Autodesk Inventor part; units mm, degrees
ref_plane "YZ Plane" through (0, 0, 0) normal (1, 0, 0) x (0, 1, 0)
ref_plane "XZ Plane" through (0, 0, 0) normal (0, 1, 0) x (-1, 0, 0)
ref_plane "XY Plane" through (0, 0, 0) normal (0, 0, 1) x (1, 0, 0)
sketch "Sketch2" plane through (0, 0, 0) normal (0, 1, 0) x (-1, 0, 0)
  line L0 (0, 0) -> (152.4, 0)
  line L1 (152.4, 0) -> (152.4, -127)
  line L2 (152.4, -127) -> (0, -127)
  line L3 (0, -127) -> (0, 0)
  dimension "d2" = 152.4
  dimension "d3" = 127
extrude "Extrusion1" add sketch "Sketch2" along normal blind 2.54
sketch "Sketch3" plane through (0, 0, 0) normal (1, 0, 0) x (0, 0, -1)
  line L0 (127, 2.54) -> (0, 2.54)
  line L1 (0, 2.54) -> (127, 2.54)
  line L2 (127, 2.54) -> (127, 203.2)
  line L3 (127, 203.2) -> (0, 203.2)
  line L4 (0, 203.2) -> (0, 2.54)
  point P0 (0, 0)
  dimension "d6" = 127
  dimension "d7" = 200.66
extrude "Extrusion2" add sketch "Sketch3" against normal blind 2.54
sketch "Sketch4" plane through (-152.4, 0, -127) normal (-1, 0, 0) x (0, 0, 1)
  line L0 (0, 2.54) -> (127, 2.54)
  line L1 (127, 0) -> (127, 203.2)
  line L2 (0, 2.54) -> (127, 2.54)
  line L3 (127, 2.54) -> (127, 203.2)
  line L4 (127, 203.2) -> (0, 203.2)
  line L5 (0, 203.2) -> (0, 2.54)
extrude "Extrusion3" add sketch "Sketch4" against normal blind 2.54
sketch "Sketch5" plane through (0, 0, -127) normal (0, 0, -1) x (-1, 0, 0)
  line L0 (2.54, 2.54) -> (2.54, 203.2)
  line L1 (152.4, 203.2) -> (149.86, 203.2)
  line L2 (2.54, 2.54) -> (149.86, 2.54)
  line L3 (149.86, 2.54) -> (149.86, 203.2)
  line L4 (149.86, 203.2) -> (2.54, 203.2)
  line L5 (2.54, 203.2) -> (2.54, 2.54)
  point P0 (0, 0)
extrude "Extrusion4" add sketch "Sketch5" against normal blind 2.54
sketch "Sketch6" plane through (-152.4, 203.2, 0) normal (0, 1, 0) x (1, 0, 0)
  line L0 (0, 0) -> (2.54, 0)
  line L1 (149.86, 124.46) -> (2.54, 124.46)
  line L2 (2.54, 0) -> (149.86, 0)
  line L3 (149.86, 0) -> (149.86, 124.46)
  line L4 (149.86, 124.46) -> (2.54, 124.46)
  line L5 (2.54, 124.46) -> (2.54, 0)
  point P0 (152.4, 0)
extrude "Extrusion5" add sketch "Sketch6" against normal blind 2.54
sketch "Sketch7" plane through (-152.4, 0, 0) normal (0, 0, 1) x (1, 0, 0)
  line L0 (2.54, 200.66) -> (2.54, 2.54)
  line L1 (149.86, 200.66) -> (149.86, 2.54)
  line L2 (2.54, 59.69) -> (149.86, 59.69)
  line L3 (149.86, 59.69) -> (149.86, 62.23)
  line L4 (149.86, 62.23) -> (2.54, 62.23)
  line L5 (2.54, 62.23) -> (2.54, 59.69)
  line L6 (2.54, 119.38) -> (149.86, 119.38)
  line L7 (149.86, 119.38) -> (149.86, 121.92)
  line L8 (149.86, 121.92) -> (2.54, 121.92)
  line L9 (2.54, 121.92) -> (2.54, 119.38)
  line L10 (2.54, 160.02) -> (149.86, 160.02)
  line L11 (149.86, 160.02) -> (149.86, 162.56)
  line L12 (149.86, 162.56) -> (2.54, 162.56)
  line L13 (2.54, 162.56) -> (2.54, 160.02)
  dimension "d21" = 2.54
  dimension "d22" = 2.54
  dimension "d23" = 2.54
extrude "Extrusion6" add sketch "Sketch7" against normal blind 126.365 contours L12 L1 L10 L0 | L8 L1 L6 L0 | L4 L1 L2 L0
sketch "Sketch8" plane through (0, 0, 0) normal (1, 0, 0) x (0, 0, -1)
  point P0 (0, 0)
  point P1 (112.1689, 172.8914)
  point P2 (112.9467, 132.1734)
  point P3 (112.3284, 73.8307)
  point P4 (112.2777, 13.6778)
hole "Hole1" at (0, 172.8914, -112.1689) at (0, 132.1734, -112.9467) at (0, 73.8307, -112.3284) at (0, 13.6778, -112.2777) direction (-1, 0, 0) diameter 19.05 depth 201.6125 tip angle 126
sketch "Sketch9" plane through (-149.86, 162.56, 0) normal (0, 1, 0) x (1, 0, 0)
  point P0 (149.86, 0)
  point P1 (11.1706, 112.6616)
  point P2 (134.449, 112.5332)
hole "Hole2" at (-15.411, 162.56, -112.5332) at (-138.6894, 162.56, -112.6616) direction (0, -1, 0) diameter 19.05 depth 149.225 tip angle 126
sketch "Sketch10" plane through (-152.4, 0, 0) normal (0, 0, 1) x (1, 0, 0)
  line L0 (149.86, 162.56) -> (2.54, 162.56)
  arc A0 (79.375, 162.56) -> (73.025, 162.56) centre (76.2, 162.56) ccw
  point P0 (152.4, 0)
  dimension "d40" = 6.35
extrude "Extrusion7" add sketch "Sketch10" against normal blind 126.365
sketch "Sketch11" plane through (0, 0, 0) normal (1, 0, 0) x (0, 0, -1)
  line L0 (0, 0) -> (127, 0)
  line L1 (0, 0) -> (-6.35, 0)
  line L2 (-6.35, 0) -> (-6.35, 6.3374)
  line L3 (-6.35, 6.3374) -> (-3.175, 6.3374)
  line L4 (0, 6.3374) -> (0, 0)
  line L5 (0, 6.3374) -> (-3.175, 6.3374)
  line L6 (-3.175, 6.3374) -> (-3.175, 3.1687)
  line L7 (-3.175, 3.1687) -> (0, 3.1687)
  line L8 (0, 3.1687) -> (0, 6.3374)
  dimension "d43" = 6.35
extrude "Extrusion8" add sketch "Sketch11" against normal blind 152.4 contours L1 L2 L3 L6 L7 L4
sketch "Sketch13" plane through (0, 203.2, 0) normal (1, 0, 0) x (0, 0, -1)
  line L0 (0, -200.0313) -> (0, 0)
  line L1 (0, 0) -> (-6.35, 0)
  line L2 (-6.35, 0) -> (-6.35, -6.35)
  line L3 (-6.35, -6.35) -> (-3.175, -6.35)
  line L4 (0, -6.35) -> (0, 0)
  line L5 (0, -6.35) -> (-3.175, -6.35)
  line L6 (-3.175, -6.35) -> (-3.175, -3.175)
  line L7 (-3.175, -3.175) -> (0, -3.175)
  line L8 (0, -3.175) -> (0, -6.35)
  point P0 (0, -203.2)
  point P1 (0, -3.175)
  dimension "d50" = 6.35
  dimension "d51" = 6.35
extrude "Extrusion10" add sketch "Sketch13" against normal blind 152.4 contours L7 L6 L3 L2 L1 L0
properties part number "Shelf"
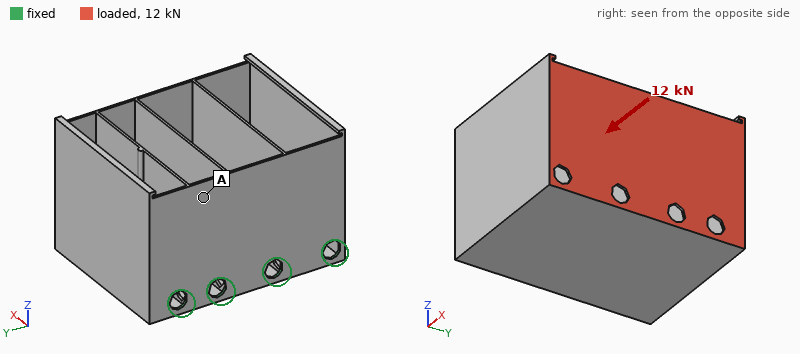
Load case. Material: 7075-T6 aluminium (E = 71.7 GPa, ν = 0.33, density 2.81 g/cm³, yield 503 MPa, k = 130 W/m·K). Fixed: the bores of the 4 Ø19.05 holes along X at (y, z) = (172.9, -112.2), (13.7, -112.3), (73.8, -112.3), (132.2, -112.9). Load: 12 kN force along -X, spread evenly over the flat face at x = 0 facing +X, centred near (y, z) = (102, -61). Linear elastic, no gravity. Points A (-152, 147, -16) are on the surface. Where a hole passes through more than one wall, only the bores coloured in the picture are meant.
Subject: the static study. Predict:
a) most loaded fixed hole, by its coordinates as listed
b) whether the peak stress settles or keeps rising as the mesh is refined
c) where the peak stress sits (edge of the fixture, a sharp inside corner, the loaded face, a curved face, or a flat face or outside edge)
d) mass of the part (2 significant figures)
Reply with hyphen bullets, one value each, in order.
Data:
- (172.9, -112.2)
- keeps rising
- edge of the fixture
- 1.2 kg
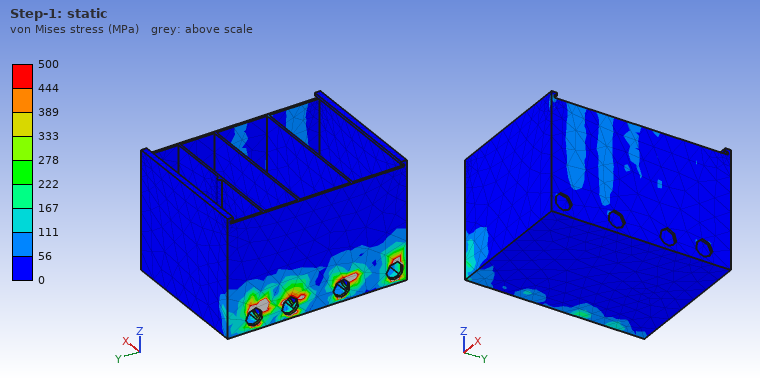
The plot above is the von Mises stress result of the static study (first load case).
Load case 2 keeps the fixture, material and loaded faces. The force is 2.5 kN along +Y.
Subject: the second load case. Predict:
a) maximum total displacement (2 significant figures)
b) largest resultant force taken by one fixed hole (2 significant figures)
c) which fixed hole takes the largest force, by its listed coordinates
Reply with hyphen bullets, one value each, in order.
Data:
- 2.6 mm
- 2.5 kN
- (13.7, -112.3)
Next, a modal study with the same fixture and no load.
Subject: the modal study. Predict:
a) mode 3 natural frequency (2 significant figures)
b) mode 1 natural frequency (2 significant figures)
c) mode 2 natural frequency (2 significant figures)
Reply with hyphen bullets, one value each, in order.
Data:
- 570 Hz
- 230 Hz
- 280 Hz
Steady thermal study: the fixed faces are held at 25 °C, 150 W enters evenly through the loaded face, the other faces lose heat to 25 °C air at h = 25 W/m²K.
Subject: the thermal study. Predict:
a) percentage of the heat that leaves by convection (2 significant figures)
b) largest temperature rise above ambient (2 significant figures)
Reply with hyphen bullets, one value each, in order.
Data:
- 85 %
- 51 K
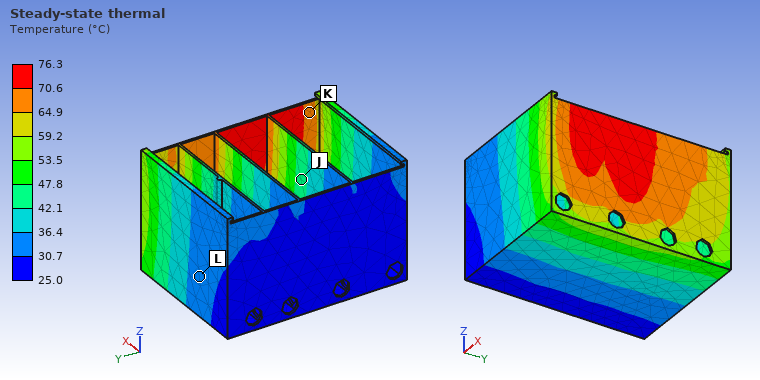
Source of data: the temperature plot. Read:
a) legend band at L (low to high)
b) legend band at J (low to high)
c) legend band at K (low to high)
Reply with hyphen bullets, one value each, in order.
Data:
- 30.7 to 36.4 °C
- 42.1 to 47.8 °C
- 64.9 to 70.6 °C
